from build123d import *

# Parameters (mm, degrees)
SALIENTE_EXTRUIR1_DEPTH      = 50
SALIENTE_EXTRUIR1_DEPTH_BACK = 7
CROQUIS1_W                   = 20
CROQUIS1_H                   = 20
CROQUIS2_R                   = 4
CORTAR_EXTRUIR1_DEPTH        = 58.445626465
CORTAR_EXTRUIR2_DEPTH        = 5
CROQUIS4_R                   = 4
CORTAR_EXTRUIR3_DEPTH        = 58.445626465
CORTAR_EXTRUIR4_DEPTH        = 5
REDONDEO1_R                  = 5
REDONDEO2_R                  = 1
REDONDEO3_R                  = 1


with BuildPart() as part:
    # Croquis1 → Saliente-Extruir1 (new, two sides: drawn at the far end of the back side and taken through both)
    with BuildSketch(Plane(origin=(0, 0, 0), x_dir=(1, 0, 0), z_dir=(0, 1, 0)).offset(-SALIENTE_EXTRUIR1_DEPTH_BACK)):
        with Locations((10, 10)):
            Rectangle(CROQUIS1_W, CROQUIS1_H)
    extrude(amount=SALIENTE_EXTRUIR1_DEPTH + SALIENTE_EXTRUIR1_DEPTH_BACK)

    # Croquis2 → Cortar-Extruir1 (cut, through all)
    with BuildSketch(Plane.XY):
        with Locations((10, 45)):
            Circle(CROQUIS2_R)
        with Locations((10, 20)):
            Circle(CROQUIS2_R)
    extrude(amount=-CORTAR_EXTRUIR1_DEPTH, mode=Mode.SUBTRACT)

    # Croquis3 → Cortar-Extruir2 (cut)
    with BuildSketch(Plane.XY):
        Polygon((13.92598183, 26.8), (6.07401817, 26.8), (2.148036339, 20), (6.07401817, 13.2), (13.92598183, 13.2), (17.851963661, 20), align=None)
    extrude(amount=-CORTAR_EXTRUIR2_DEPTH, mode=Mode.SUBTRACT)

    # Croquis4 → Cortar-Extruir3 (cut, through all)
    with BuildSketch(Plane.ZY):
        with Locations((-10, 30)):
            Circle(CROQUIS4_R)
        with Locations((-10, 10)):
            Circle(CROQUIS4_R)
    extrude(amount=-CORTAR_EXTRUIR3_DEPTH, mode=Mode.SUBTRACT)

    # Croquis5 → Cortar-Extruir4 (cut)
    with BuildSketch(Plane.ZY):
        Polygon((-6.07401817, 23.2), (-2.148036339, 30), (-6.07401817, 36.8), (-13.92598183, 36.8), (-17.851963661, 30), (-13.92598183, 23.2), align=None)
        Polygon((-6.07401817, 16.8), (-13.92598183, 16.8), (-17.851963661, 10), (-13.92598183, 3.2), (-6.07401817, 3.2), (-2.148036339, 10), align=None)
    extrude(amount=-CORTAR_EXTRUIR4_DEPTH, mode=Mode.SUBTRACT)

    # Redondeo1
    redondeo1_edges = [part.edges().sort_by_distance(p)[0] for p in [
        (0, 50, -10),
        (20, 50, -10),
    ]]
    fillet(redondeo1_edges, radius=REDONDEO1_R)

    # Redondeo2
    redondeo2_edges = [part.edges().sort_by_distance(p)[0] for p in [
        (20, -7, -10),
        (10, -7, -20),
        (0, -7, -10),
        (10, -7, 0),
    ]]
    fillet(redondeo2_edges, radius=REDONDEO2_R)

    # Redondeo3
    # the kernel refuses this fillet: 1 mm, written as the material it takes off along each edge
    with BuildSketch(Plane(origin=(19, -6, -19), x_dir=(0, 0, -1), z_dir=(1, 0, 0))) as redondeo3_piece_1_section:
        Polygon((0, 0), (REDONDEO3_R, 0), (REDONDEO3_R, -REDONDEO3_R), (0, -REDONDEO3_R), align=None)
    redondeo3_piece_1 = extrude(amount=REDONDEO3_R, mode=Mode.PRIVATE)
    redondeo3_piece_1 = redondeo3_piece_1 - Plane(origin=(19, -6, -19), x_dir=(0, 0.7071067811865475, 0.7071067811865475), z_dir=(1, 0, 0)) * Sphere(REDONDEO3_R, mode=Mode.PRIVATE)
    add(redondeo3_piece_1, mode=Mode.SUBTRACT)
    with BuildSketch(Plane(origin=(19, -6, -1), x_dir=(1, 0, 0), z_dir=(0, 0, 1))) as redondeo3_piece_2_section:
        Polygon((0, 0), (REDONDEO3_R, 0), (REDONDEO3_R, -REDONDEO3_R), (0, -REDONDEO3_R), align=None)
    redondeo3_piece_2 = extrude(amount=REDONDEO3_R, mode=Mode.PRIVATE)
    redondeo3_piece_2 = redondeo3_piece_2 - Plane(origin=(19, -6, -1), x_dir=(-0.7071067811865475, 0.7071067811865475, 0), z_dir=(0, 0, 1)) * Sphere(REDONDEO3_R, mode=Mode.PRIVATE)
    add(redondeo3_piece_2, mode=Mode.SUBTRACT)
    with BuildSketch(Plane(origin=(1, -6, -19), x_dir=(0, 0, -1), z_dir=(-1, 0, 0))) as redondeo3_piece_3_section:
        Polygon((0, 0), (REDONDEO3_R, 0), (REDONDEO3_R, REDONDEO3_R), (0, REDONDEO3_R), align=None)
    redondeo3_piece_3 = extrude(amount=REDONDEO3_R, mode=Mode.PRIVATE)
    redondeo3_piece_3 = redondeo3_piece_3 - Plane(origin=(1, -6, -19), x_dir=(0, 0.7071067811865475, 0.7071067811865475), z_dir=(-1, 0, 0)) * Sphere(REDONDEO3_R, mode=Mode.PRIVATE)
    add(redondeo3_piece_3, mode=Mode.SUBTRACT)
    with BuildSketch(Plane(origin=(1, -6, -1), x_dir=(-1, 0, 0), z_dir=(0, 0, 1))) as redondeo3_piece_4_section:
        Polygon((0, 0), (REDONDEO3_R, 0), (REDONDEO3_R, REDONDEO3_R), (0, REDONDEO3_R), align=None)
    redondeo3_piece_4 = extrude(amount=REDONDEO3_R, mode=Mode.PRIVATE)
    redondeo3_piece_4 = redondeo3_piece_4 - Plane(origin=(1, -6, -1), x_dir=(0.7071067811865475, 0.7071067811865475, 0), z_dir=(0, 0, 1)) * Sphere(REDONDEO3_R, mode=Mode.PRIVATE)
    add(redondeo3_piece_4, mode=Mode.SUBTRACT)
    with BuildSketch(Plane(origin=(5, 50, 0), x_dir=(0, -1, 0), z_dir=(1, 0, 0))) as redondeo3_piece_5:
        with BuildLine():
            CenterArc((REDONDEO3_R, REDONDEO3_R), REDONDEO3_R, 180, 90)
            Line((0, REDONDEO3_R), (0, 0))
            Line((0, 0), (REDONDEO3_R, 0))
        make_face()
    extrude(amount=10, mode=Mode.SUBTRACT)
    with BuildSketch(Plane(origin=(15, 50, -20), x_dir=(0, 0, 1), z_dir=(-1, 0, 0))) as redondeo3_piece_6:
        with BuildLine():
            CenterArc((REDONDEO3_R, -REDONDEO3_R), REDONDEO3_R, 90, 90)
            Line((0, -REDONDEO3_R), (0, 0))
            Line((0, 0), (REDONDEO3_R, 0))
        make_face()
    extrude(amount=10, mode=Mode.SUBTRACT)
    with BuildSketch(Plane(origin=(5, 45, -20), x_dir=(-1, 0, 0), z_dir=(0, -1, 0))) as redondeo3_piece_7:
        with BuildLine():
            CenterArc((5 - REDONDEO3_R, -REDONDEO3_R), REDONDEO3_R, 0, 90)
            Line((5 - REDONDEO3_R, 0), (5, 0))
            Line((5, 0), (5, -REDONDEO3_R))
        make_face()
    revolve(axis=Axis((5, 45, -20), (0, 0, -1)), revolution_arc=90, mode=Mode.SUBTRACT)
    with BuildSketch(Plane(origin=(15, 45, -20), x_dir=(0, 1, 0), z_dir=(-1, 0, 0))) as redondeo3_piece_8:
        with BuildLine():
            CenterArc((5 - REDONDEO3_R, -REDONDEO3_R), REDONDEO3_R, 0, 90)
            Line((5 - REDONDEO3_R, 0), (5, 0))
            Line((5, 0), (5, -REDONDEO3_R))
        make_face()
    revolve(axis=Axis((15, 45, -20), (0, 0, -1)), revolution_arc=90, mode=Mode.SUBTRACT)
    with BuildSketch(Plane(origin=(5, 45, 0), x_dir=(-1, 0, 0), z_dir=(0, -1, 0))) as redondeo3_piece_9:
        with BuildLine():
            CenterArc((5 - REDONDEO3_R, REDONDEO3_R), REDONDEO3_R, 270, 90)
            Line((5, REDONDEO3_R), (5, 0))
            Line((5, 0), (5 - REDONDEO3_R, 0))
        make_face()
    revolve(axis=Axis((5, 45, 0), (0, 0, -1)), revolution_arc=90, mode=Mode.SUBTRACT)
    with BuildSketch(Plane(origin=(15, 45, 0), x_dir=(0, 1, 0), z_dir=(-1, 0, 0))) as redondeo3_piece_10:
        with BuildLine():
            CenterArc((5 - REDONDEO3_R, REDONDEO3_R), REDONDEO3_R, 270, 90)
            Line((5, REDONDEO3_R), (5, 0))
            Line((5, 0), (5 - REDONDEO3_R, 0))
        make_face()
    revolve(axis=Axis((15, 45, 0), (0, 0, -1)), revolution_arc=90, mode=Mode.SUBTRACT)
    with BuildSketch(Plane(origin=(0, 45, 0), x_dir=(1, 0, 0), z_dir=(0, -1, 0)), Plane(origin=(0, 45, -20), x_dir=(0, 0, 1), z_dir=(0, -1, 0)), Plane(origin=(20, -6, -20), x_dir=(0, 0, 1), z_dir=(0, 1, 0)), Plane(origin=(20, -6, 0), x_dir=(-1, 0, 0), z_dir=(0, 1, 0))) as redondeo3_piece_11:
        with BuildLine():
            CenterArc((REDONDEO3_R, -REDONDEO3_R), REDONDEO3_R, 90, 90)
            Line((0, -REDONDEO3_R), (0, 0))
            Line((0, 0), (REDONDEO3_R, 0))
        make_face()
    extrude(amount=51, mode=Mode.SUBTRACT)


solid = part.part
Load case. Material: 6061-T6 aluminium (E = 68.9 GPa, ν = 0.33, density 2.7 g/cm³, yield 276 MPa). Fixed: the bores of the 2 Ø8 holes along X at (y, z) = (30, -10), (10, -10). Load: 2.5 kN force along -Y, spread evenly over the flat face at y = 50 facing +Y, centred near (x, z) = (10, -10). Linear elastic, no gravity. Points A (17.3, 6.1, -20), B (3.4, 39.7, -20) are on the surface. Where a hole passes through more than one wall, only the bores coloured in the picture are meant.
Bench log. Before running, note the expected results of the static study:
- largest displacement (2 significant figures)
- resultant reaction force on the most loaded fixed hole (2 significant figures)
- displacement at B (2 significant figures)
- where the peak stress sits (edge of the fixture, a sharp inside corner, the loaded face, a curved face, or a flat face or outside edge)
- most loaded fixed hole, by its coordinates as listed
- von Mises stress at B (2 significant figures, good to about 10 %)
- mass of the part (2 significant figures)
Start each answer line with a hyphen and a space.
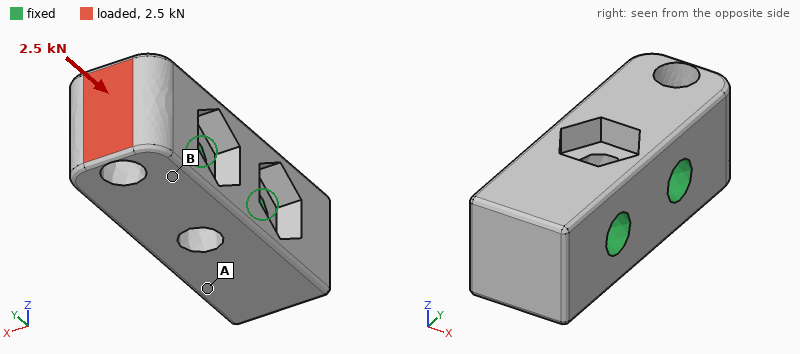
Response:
- 13 µm
- 2.3 kN
- 3.2 µm
- the loaded face
- (30, -10)
- 16 MPa
- 45 g
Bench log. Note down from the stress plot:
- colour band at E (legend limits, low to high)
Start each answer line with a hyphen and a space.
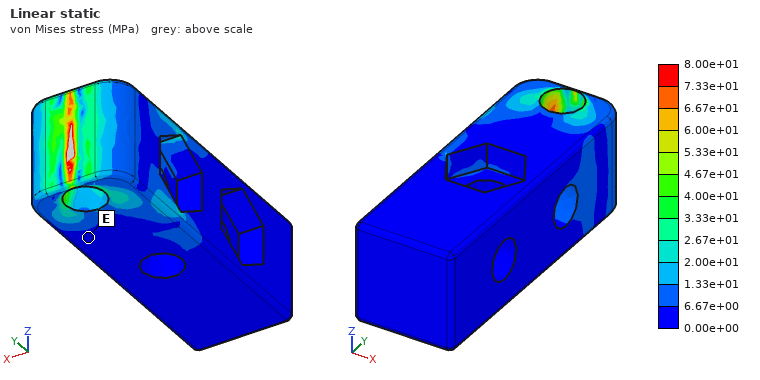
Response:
- 0.00e+00 to 6.67e+00 MPa
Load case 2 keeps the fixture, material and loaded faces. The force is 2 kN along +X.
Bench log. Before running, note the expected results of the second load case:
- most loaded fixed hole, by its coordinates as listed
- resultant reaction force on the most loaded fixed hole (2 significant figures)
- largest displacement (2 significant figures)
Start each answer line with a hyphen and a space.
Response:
- (30, -10)
- 2.2 kN
- 23 µm
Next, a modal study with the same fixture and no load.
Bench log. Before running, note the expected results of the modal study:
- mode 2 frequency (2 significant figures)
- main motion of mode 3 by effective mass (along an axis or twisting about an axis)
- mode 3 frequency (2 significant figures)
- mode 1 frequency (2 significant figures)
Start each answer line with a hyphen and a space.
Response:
- 24 kHz
- along Z
- 27 kHz
- 24 kHz
